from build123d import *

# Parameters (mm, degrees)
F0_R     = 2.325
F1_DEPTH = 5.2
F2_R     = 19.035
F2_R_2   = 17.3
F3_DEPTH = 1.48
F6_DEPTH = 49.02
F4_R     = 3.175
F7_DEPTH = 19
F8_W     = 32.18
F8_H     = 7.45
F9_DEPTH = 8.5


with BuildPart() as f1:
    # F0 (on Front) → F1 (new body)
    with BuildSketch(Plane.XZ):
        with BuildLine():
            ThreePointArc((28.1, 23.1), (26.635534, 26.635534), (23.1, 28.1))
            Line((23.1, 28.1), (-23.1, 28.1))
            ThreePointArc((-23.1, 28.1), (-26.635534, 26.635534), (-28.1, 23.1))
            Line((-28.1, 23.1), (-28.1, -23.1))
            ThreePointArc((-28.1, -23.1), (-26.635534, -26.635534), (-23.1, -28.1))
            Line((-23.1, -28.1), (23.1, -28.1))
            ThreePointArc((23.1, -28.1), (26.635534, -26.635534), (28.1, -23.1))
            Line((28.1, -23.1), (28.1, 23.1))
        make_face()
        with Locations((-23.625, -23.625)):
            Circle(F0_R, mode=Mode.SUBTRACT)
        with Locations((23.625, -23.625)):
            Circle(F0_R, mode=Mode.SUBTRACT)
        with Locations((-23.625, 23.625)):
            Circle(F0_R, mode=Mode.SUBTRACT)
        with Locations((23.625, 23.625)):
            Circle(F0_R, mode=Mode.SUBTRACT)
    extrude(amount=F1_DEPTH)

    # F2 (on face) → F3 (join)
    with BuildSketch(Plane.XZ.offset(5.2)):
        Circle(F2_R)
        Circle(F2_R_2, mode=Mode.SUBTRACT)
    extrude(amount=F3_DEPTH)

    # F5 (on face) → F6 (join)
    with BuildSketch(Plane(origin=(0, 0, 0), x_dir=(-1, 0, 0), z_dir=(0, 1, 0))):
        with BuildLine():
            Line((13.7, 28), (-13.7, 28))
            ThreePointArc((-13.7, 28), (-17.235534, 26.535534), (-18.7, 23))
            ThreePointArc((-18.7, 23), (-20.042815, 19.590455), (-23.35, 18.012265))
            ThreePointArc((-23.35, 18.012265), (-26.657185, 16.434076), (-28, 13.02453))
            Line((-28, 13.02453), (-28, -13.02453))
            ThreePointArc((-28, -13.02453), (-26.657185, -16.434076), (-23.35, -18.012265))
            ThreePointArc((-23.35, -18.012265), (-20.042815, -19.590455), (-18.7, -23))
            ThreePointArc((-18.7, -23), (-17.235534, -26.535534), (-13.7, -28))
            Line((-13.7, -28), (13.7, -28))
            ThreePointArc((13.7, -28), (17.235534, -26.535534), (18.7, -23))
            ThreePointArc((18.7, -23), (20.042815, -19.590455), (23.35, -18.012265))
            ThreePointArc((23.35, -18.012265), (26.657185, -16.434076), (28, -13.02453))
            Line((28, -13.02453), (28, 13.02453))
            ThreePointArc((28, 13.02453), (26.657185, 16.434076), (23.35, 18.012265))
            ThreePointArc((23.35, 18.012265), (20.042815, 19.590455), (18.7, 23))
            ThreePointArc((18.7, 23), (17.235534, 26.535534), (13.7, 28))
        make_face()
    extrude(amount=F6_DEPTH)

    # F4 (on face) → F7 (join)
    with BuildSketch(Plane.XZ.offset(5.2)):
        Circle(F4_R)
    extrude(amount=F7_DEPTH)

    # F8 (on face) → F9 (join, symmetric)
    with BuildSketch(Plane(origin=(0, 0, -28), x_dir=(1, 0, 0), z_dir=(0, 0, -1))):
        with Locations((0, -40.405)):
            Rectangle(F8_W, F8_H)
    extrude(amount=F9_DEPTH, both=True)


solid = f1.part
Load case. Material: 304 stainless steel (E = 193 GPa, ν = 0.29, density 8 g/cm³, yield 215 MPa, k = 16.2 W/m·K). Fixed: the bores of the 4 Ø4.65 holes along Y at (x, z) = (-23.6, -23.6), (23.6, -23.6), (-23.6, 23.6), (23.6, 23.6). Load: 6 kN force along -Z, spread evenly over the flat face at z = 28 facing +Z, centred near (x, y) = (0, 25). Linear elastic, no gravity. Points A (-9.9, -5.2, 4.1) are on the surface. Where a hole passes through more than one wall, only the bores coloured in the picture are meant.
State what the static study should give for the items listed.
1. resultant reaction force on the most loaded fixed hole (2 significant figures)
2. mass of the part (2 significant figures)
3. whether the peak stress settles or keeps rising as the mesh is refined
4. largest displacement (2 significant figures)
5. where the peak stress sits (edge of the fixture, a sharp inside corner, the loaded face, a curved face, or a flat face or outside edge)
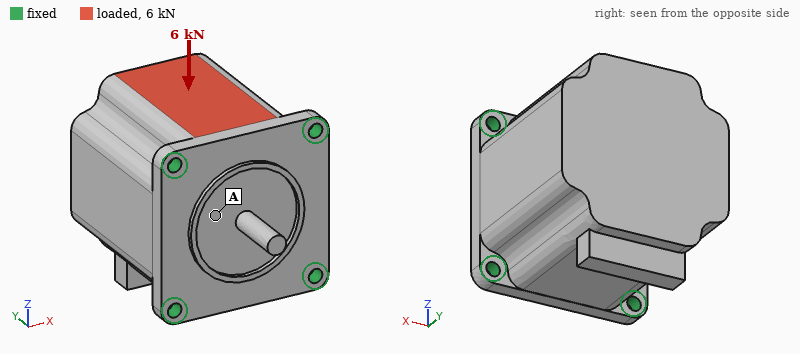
2.5 kN
1.2 kg
keeps rising
11 µm
edge of the fixture
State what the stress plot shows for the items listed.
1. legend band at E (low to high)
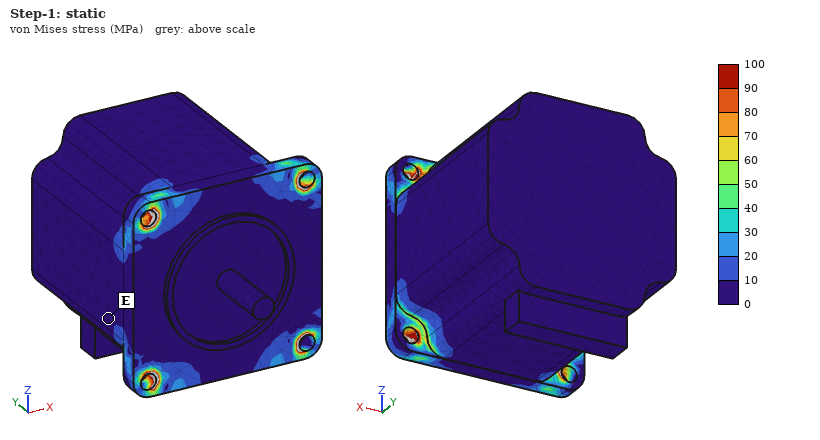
0 to 10 MPa
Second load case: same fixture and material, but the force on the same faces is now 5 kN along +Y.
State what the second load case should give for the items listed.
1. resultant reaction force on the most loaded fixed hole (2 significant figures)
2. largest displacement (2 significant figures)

3.0 kN
11 µm
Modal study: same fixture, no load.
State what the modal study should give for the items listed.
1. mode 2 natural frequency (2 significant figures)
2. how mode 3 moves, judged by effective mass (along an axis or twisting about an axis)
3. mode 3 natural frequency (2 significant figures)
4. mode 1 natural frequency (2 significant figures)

4100 Hz
along Y
6500 Hz
4100 Hz
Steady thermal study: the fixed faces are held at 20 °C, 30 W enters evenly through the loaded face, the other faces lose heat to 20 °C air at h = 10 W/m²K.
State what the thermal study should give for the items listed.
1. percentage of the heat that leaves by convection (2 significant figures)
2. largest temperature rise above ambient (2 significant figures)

21 %
67 K
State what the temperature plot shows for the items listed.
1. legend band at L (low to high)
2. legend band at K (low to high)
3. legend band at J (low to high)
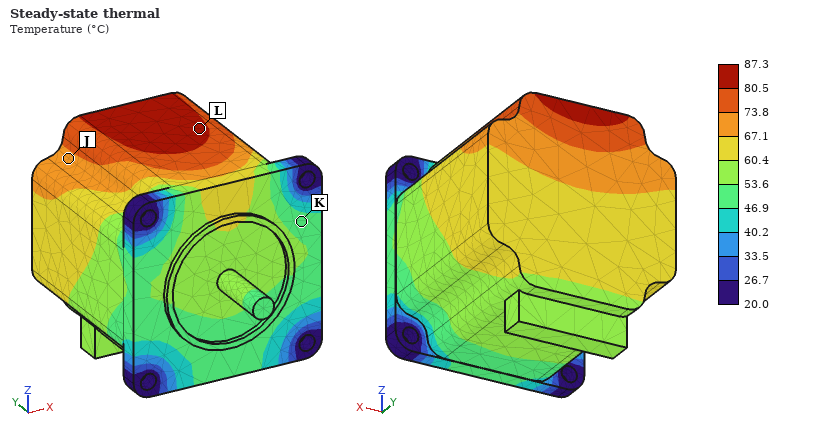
80.5 to 87.3 °C
46.9 to 53.6 °C
67.1 to 73.8 °C
